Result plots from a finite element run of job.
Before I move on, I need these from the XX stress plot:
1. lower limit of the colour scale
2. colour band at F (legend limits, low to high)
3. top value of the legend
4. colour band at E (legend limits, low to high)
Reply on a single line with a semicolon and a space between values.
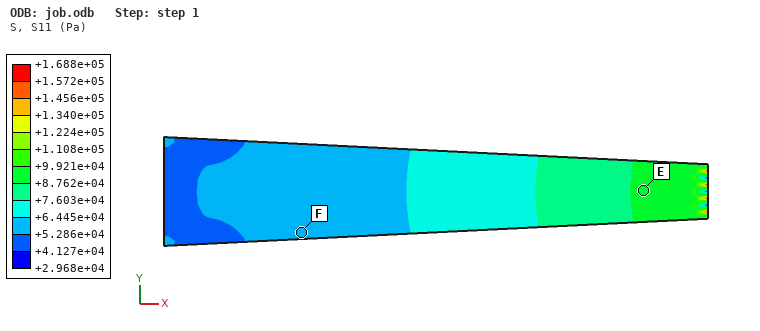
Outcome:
+2.968e+04 Pa; +5.286e+04 to +6.445e+04 Pa; +1.688e+05 Pa; +8.762e+04 to +9.921e+04 Pa
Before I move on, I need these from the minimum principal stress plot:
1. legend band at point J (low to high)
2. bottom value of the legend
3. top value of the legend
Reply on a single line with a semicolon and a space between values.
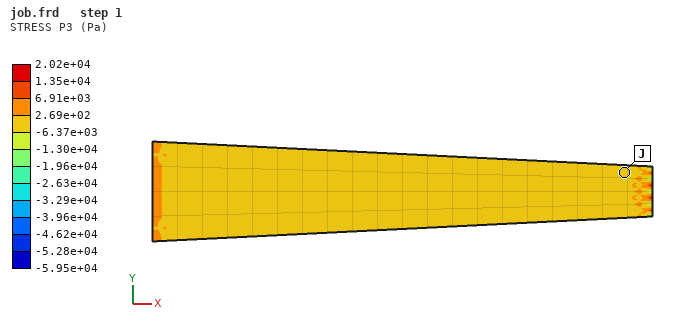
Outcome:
-6.37e+03 to 2.69e+02 Pa; -5.95e+04 Pa; 2.02e+04 Pa
